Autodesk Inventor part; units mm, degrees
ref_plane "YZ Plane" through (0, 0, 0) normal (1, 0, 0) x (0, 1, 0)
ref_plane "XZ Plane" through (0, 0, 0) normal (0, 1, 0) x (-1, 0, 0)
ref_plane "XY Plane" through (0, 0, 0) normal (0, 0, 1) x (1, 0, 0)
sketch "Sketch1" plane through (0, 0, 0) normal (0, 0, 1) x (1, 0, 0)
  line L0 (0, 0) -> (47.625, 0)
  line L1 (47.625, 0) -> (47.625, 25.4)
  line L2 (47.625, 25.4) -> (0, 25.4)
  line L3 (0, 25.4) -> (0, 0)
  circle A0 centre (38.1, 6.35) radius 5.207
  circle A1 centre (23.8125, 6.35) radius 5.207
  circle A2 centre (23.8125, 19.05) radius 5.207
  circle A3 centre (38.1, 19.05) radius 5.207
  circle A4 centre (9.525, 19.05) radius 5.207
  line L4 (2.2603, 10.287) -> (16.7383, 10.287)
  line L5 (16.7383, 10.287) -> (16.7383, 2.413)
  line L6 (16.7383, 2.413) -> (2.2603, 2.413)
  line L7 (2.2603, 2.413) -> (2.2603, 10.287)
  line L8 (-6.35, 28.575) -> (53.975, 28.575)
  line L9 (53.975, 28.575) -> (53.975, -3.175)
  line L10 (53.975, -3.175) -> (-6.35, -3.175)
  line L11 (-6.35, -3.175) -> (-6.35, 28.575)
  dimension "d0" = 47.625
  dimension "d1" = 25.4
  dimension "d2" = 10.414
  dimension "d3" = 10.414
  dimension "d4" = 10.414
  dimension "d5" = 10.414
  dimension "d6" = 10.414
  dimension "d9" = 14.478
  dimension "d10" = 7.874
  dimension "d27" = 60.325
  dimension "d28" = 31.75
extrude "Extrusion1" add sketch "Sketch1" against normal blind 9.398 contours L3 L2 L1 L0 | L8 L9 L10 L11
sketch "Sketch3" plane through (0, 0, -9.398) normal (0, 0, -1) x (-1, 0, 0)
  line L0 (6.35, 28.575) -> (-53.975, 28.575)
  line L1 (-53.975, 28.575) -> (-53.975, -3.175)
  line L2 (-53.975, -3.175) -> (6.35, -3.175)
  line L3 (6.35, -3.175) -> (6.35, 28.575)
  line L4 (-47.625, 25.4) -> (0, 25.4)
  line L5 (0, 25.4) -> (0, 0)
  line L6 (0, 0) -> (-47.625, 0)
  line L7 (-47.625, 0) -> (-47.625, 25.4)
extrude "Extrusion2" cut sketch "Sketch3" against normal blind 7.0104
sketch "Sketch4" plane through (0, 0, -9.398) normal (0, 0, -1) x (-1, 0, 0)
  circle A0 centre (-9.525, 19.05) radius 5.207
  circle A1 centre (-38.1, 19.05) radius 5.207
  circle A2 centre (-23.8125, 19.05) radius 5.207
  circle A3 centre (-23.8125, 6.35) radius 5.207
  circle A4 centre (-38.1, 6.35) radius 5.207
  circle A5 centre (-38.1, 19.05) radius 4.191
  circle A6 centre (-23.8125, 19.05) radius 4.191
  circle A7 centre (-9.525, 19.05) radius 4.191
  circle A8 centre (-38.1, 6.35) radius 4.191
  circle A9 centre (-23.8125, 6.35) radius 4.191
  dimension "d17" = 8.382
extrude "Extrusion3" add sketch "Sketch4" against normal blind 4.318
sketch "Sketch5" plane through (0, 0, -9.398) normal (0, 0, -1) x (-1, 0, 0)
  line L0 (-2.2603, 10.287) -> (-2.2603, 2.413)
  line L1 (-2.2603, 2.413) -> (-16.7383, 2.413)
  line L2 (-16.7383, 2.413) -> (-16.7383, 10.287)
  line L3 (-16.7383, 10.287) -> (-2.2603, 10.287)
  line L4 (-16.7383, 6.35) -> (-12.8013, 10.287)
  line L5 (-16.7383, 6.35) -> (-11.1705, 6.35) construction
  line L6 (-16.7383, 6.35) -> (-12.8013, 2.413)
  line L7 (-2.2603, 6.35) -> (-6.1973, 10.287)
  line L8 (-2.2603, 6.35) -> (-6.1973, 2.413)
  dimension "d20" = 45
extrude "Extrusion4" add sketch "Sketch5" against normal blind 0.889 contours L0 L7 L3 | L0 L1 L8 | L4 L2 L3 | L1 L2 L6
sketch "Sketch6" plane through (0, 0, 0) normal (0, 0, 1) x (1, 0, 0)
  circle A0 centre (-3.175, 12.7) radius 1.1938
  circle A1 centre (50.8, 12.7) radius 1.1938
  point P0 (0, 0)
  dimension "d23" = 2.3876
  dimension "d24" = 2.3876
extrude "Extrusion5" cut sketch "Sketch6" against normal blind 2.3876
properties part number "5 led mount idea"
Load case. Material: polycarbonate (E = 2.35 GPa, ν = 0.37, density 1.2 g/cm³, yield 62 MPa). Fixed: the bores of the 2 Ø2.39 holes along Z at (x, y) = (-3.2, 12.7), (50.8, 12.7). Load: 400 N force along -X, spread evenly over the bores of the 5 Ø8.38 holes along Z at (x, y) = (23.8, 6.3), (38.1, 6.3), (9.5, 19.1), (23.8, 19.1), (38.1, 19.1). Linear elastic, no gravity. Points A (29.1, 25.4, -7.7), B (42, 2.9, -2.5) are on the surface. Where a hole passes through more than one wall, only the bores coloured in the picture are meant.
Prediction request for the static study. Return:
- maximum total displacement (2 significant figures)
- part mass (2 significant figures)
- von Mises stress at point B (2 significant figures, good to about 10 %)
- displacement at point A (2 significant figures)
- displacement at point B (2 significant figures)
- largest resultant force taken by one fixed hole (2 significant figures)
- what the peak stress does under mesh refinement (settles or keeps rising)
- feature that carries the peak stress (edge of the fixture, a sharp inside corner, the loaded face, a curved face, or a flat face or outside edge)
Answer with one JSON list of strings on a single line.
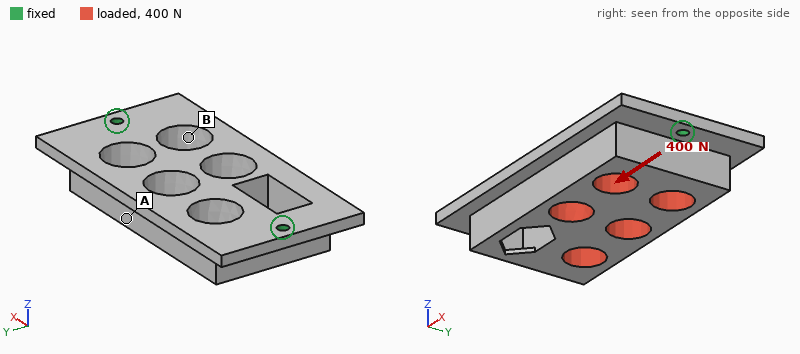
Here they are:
["71 µm", "10 g", "2.4 MPa", "58 µm", "50 µm", "210 N", "keeps rising", "edge of the fixture"]
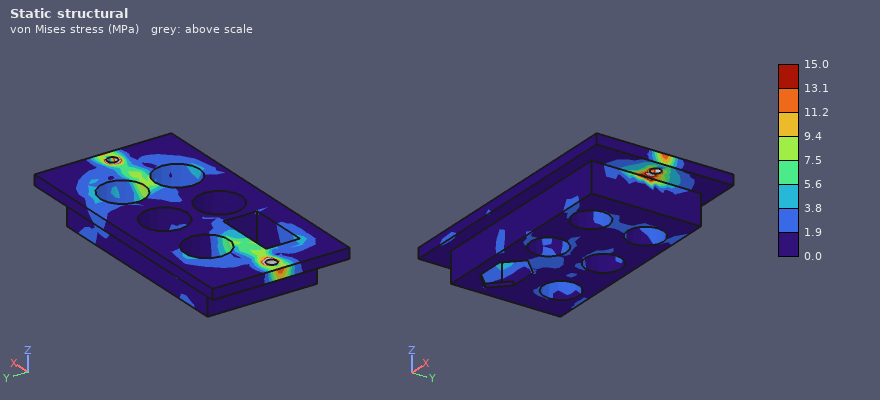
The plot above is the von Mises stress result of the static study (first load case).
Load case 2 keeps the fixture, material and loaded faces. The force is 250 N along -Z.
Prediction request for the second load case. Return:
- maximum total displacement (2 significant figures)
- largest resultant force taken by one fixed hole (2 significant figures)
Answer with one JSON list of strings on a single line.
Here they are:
["0.41 mm", "200 N"]
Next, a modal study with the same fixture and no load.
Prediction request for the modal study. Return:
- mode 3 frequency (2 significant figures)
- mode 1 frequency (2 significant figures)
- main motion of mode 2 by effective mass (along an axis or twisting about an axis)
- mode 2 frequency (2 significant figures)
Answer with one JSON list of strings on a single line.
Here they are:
["2800 Hz", "930 Hz", "along Z", "2000 Hz"]
